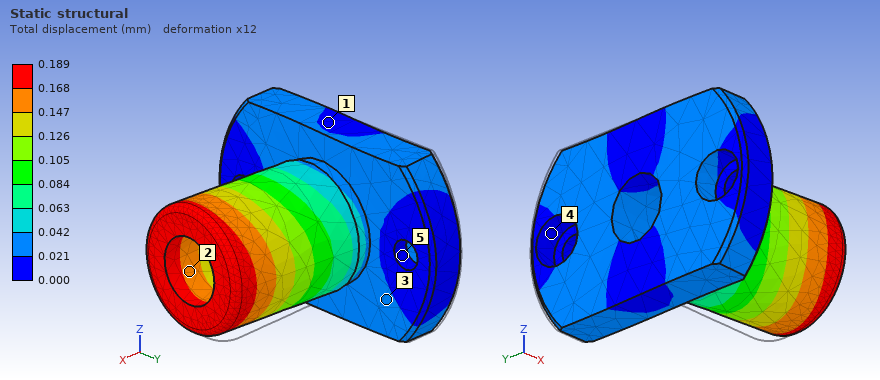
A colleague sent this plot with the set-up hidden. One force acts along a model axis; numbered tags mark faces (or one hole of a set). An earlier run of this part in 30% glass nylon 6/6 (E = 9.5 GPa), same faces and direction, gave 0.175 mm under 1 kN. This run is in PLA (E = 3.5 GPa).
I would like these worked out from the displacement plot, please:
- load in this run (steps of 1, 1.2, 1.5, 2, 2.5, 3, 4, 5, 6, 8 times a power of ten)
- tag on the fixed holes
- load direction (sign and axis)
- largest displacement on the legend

400 N
5
-Y
0.189 mm
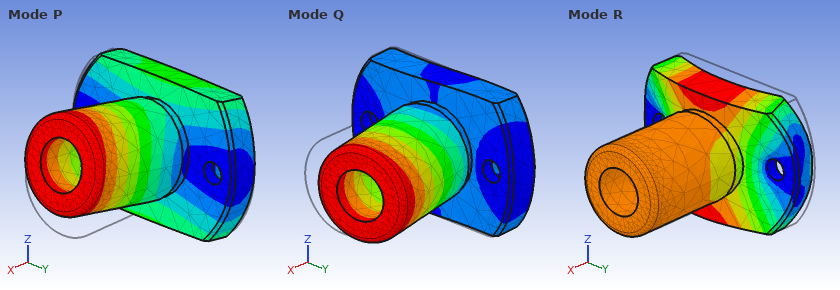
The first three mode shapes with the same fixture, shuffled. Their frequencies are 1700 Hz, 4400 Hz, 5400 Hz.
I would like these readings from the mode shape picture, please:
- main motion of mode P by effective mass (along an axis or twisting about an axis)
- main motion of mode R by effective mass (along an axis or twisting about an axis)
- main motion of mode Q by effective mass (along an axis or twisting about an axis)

along Z
along X
along Y
